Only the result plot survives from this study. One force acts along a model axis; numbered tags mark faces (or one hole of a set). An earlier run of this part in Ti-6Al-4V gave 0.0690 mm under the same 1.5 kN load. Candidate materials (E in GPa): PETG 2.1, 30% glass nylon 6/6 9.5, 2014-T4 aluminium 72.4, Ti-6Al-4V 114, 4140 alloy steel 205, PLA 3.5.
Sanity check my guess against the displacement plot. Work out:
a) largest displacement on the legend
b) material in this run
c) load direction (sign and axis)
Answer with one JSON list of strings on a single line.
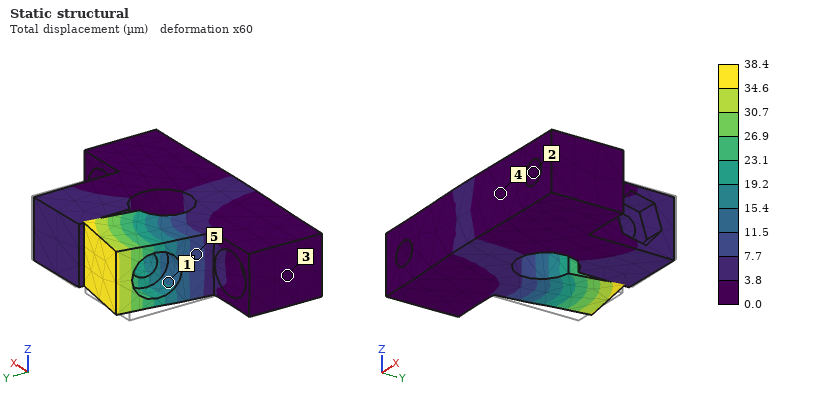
["38.4 µm", "4140 alloy steel", "+X"]
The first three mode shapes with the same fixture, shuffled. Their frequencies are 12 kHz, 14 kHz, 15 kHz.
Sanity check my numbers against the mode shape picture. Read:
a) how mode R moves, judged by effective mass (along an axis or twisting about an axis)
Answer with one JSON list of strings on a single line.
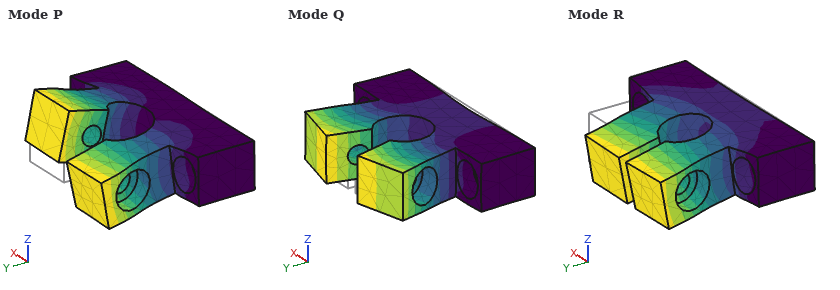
["along Z"]
